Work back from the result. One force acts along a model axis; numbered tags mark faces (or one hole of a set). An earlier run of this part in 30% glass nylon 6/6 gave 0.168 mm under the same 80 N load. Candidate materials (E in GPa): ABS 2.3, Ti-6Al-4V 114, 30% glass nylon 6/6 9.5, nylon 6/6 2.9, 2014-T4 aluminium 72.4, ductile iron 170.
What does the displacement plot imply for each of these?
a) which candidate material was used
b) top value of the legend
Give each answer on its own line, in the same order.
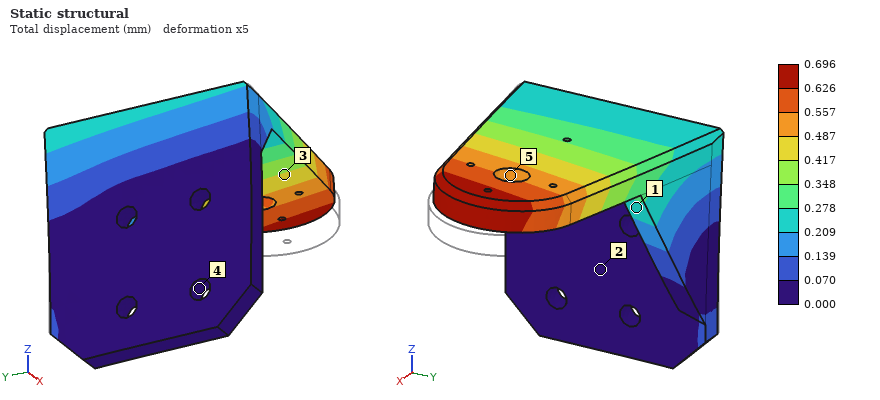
ABS
0.696 mm
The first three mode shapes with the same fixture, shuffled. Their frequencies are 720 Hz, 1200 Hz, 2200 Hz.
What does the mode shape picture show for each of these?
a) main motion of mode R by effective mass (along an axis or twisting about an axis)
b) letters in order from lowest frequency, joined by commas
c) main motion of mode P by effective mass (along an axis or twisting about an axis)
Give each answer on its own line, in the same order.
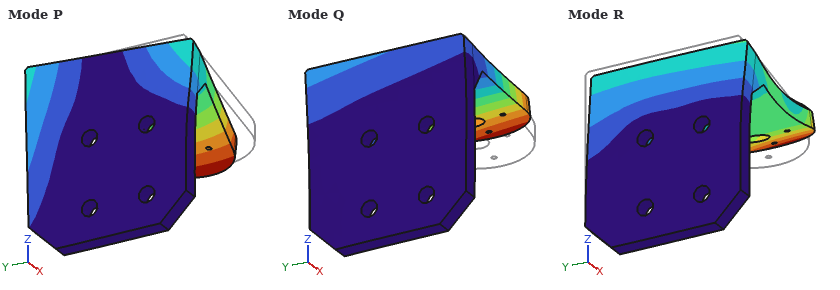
along X
Q, P, R
along Y
